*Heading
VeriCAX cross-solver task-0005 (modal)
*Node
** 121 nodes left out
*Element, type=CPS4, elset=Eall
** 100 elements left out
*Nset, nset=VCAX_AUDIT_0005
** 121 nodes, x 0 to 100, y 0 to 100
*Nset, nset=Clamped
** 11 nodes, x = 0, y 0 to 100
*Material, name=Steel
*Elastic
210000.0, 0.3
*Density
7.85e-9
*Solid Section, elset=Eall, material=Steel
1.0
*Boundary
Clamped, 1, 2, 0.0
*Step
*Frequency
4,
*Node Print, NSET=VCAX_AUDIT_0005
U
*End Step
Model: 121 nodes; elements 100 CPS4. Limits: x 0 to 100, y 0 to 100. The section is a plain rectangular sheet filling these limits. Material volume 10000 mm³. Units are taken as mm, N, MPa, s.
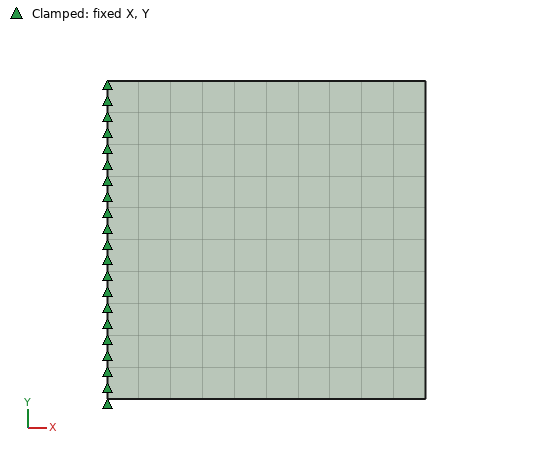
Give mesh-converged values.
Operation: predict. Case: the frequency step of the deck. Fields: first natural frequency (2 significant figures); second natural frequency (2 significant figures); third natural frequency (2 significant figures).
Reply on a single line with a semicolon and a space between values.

5400 Hz; 13000 Hz; 15000 Hz
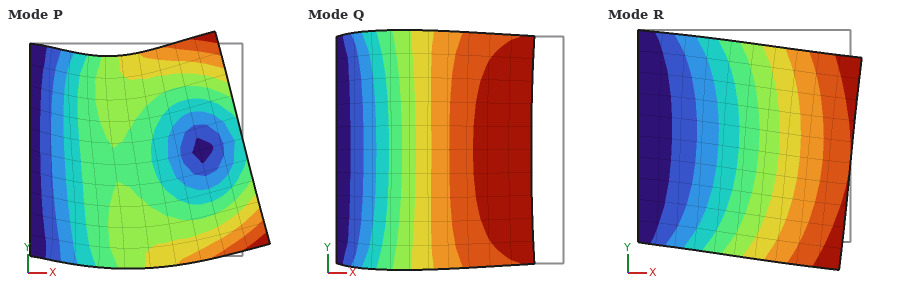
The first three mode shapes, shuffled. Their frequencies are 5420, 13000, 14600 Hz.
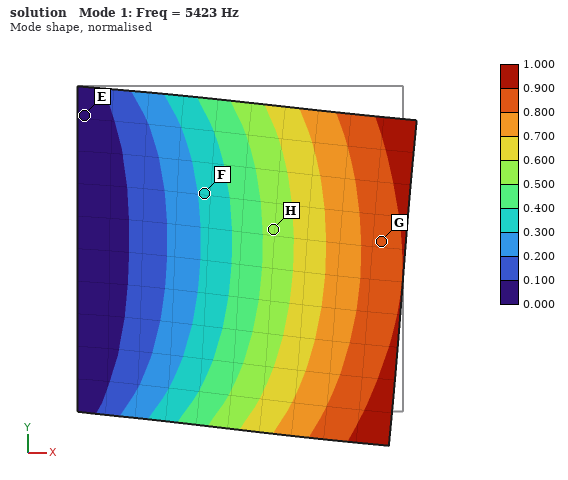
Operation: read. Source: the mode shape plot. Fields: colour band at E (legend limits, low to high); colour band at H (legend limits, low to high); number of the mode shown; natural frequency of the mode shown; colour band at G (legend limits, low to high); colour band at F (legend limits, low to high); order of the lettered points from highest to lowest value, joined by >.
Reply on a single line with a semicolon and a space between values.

0.000 to 0.100; 0.500 to 0.600; 1; 5423 Hz; 0.800 to 0.900; 0.300 to 0.400; G > H > F > E
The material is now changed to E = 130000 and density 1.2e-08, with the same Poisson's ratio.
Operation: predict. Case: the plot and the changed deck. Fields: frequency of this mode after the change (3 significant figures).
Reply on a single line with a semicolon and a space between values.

3450 Hz
